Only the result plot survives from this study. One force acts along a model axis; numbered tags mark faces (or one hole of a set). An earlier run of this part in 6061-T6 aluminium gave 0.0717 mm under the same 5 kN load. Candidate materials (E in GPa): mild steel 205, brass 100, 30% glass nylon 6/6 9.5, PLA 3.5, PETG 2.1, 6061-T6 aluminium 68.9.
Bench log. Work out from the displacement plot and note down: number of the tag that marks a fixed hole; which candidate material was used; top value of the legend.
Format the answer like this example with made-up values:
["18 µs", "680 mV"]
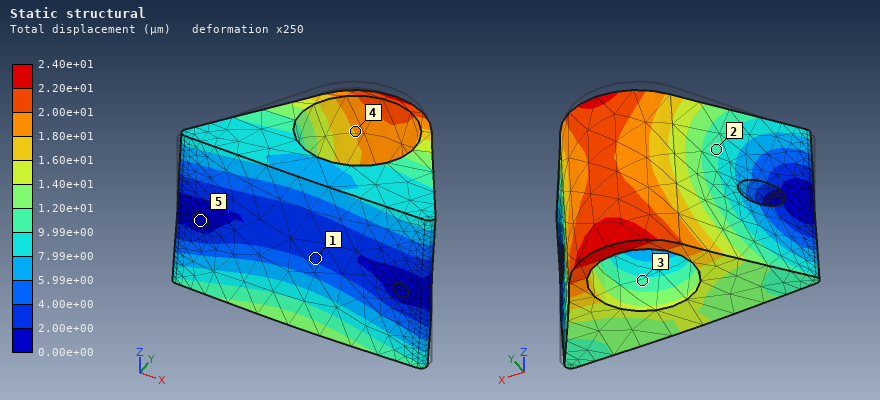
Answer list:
["5", "mild steel", "2.40e+01 µm"]
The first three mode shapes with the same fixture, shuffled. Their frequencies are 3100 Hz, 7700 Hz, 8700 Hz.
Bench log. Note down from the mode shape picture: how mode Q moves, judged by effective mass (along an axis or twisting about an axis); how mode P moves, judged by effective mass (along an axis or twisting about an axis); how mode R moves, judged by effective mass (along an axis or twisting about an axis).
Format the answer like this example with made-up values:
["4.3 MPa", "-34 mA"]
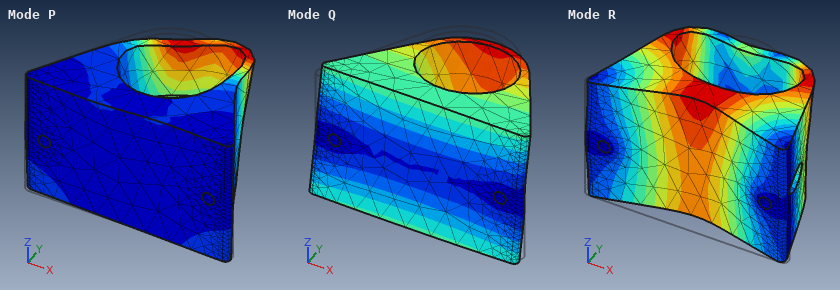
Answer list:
["along Z", "along X", "along Y"]
